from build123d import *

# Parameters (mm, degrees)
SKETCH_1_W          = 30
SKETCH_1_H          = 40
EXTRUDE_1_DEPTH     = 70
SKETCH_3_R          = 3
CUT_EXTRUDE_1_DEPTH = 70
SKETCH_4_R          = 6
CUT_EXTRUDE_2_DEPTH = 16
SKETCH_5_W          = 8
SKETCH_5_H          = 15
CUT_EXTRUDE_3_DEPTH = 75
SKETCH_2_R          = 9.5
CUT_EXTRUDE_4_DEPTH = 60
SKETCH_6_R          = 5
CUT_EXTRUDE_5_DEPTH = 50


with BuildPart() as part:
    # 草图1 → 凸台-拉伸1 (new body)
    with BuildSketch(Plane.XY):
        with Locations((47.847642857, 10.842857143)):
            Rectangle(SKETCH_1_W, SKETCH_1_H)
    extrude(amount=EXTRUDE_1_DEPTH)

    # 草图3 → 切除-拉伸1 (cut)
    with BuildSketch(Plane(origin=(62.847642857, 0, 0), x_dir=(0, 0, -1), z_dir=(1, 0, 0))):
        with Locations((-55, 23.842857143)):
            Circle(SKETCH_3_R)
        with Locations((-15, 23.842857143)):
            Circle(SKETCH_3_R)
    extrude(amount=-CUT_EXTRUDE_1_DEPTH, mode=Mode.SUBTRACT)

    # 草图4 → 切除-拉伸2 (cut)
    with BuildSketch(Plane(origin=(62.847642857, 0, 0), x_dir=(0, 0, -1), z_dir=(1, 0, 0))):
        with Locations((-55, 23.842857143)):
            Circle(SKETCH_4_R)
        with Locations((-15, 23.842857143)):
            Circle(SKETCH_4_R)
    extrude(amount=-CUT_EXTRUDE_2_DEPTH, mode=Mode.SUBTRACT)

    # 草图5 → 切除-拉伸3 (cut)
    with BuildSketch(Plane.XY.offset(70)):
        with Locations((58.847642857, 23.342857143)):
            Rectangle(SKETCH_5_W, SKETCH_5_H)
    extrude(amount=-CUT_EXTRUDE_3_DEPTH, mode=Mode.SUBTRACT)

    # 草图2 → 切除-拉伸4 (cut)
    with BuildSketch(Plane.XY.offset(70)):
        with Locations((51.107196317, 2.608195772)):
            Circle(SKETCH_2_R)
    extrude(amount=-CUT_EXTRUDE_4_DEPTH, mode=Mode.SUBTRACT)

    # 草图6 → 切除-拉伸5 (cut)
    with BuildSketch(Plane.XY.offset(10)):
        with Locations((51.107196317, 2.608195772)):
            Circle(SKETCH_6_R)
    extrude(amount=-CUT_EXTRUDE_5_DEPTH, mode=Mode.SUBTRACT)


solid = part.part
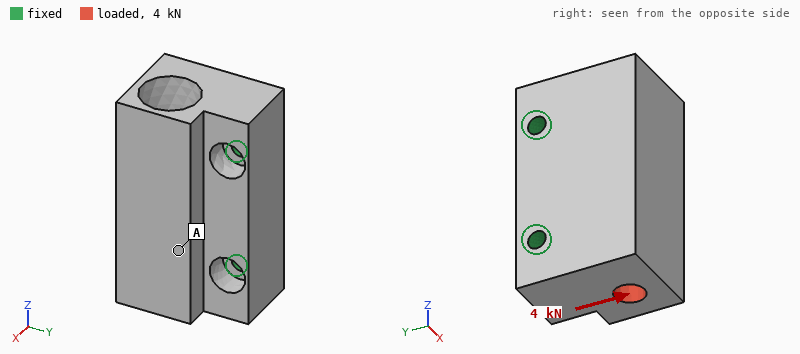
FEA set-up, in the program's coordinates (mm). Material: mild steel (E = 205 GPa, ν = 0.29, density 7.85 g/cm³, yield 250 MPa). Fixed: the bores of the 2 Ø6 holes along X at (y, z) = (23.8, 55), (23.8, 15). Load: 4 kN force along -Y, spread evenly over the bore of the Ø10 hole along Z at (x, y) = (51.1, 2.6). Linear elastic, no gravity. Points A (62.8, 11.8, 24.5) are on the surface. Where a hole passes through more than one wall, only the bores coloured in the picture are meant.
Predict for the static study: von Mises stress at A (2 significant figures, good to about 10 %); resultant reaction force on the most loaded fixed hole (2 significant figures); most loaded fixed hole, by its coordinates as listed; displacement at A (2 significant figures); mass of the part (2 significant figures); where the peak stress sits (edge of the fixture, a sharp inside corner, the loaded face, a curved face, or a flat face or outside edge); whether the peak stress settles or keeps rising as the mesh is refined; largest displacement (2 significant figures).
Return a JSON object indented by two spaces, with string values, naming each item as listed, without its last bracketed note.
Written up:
{
  "von Mises stress at A": "6.0 MPa",
  "resultant reaction force on the most loaded fixed hole": "4.7 kN",
  "most loaded fixed hole, by its coordinates as listed": "(23.8, 15)",
  "displacement at A": "6.2 µm",
  "mass of the part": "430 g",
  "where the peak stress sits": "edge of the fixture",
  "whether the peak stress settles or keeps rising as the mesh is refined": "keeps rising",
  "largest displacement": "12 µm"
}
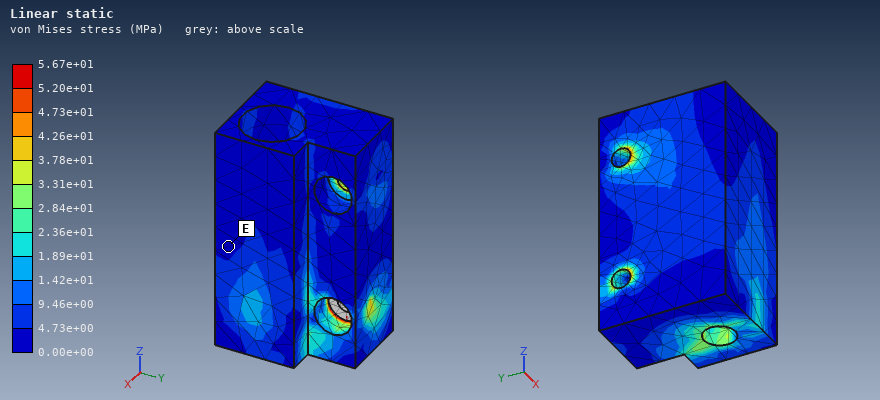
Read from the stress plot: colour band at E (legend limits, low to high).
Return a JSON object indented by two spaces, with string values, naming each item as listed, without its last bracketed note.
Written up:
{
  "colour band at E": "0.00e+00 to 4.73e+00 MPa"
}
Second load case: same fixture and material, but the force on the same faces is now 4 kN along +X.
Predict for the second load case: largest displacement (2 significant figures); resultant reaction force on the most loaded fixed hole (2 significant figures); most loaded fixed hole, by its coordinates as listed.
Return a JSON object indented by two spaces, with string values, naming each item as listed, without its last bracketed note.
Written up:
{
  "largest displacement": "20 µm",
  "resultant reaction force on the most loaded fixed hole": "4.4 kN",
  "most loaded fixed hole, by its coordinates as listed": "(23.8, 15)"
}
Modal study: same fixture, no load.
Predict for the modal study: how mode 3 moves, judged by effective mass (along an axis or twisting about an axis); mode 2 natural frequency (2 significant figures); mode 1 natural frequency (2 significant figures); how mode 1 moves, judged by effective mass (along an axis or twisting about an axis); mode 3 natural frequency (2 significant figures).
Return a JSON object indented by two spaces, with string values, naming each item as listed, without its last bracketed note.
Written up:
{
  "how mode 3 moves, judged by effective mass": "along Z",
  "mode 2 natural frequency": "12 kHz",
  "mode 1 natural frequency": "6000 Hz",
  "how mode 1 moves, judged by effective mass": "along X",
  "mode 3 natural frequency": "13 kHz"
}
